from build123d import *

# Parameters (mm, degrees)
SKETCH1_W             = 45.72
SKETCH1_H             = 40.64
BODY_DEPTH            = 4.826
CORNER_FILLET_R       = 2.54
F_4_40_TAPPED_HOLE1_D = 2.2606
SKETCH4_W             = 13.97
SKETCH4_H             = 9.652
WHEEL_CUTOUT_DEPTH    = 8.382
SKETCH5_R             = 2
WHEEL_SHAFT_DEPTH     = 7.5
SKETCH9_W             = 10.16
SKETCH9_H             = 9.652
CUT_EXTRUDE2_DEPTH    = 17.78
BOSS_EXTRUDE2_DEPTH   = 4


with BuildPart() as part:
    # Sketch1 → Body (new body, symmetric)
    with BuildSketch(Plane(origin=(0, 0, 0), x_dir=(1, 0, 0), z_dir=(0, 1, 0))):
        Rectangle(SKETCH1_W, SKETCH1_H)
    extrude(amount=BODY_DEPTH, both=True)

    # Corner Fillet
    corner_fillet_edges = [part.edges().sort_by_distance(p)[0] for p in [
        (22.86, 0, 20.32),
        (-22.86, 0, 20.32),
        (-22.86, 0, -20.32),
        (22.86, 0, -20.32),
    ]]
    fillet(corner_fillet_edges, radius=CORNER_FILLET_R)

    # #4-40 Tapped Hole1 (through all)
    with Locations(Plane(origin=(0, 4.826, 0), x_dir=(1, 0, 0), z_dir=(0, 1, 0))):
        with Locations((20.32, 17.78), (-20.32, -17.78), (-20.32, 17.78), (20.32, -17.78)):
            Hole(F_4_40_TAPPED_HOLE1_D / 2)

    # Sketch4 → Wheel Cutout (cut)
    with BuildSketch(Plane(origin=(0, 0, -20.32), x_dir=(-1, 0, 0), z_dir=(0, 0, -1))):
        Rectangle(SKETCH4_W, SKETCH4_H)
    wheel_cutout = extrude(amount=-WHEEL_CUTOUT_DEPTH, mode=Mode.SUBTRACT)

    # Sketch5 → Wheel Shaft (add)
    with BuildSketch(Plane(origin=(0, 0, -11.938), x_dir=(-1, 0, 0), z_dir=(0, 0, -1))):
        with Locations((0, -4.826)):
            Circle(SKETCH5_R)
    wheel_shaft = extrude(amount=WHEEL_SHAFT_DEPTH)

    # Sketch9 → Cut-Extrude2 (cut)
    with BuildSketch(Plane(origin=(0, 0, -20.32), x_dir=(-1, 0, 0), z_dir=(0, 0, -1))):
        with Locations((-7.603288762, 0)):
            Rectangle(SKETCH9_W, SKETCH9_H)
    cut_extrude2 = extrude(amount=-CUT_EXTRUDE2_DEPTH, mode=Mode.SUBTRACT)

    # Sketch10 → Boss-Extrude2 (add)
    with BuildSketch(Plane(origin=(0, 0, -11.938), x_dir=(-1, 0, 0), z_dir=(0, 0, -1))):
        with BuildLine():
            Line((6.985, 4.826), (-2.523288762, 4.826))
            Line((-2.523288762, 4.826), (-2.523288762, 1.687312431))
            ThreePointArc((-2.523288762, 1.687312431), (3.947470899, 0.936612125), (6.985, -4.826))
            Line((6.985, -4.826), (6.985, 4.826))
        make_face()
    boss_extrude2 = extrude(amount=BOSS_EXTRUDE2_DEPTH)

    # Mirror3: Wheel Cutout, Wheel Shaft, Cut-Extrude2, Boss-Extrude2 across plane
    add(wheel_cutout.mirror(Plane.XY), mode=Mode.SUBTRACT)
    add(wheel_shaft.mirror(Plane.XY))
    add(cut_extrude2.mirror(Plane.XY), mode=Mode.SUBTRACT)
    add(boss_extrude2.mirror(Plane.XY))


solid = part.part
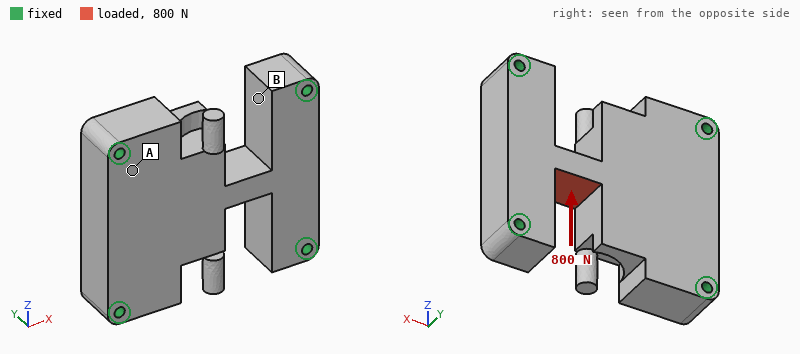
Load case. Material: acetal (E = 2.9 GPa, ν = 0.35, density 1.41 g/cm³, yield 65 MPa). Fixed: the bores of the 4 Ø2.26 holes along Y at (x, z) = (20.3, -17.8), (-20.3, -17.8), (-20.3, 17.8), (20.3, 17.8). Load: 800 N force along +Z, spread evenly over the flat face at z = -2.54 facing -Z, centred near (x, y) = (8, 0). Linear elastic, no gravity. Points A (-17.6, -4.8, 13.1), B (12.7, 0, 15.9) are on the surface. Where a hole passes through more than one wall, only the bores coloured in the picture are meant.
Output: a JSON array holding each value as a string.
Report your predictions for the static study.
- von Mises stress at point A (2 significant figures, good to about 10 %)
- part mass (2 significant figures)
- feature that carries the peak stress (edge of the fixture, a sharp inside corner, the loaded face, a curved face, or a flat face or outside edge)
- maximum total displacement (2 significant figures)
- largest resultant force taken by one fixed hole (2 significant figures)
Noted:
["3.2 MPa", "19 g", "a flat face or outside edge", "88 µm", "310 N"]
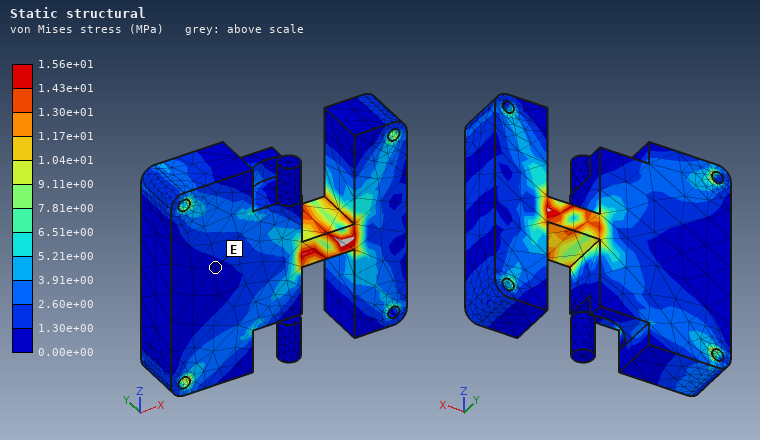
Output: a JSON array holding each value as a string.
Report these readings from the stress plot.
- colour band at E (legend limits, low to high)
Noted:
["0.00e+00 to 1.30e+00 MPa"]
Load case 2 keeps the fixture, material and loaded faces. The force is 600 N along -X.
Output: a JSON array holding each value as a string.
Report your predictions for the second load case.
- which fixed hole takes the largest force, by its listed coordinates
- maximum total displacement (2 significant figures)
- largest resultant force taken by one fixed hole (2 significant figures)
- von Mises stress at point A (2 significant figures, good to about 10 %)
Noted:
["(-20.3, 17.8)", "59 µm", "300 N", "3.5 MPa"]
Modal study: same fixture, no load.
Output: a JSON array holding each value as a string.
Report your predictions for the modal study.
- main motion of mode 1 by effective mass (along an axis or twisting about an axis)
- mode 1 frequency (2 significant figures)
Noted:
["along Y", "3600 Hz"]
